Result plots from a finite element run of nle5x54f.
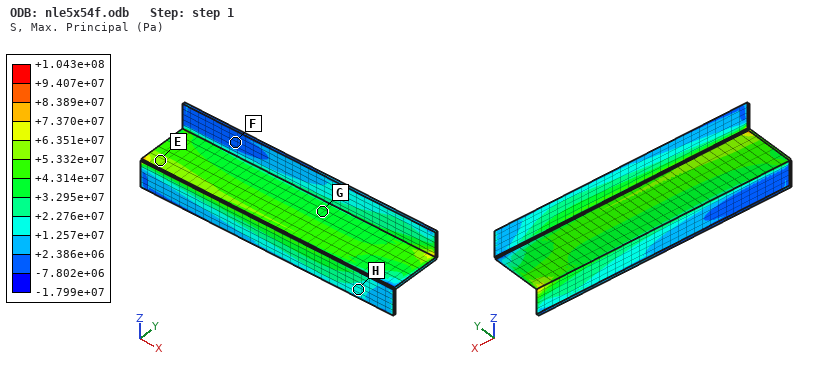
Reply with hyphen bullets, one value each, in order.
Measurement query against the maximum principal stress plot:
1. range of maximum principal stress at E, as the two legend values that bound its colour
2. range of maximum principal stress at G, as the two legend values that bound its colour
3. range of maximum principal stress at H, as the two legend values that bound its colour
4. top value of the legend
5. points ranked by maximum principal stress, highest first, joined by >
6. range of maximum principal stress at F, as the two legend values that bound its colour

- +5.332e+07 to +6.351e+07 Pa
- +3.295e+07 to +4.314e+07 Pa
- +1.257e+07 to +2.276e+07 Pa
- +1.043e+08 Pa
- E > G > H > F
- -7.802e+06 to +2.386e+06 Pa
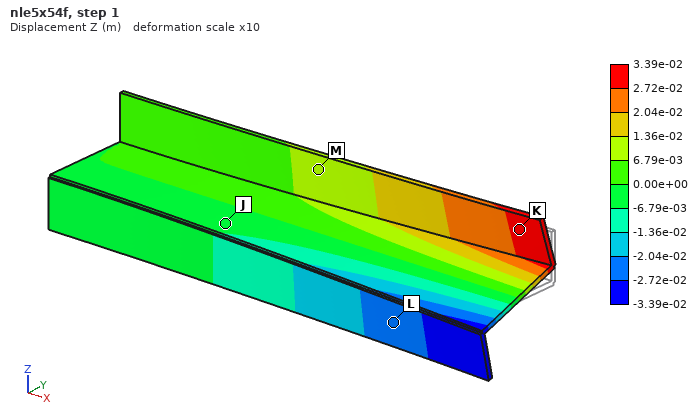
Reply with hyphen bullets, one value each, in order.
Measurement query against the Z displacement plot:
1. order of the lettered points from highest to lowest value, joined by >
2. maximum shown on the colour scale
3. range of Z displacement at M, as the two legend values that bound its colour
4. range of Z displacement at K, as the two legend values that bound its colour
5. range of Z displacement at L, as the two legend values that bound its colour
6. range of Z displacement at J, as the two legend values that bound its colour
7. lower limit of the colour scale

- K > M > J > L
- 3.39e-02 m
- 6.79e-03 to 1.36e-02 m
- 2.72e-02 to 3.39e-02 m
- -2.72e-02 to -2.04e-02 m
- -6.79e-03 to 0.00e+00 m
- -3.39e-02 m
